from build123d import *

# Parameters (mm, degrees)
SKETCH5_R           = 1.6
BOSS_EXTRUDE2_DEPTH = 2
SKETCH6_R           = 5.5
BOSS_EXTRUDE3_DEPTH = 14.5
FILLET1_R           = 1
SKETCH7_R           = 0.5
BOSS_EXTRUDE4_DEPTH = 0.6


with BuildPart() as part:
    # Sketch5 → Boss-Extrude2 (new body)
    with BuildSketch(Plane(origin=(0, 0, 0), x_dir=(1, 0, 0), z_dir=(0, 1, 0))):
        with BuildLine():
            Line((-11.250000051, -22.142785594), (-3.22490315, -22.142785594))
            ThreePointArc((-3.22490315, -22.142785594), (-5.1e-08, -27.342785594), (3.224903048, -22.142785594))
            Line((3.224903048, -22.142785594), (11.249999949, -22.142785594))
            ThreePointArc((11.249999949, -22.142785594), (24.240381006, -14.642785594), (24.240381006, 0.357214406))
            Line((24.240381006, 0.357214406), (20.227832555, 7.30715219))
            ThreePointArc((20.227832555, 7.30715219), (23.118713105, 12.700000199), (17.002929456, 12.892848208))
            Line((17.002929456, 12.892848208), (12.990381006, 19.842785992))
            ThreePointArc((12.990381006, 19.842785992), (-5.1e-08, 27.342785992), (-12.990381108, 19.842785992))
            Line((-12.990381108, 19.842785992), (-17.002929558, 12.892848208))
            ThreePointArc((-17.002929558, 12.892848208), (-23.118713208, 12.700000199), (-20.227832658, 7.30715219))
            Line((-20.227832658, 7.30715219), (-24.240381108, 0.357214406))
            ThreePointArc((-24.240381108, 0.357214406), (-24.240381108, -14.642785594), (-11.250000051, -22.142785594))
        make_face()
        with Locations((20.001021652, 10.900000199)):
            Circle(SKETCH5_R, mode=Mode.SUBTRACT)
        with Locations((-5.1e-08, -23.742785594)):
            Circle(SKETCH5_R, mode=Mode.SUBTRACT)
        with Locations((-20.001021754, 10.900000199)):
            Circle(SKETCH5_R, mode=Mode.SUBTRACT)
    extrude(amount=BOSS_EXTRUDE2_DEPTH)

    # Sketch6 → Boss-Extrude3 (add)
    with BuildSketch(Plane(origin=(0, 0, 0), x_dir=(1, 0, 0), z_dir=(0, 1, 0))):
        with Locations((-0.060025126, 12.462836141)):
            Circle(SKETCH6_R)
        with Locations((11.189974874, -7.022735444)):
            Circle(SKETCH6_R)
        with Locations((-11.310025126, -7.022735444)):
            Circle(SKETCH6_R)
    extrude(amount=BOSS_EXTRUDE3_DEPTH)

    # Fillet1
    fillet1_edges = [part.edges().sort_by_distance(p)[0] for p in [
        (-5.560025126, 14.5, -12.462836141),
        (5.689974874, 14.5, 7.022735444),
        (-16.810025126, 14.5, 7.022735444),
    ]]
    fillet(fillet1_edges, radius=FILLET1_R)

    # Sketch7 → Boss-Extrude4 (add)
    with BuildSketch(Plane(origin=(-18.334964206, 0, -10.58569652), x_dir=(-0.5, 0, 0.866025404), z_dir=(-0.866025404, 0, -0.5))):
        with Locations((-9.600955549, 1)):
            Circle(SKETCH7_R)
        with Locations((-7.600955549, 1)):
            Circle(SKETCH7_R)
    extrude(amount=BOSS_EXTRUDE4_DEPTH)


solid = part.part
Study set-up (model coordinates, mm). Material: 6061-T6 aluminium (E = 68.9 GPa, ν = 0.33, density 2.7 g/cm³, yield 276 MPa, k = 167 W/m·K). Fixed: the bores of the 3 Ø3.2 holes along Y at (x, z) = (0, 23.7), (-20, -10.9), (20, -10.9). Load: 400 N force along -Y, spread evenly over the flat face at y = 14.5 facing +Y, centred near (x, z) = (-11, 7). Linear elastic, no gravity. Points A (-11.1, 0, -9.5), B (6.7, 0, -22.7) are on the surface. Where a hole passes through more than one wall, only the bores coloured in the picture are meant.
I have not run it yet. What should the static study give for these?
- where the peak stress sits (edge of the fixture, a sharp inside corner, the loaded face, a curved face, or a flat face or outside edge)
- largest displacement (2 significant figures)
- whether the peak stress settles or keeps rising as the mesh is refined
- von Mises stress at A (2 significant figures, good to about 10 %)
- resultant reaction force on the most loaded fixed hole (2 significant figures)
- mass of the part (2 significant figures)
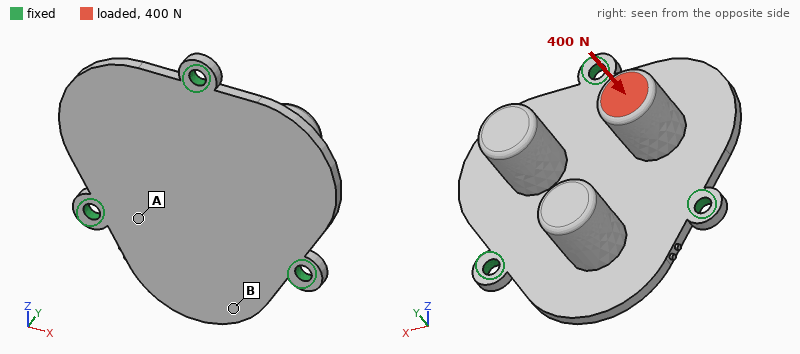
edge of the fixture
0.19 mm
keeps rising
37 MPa
210 N
20 g
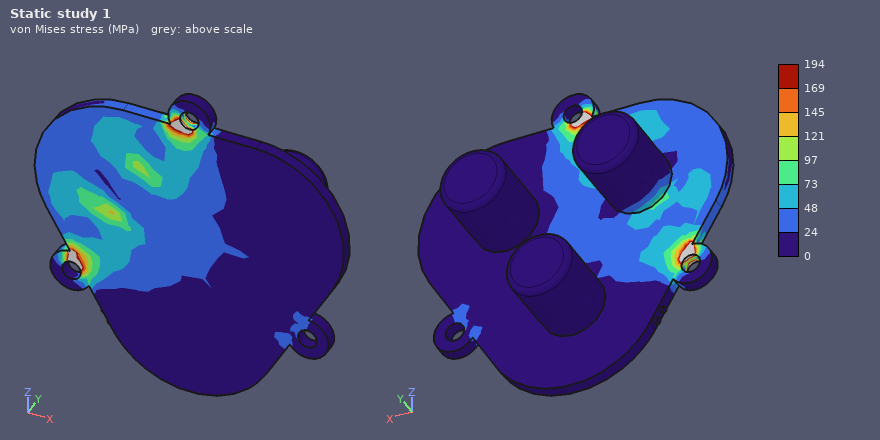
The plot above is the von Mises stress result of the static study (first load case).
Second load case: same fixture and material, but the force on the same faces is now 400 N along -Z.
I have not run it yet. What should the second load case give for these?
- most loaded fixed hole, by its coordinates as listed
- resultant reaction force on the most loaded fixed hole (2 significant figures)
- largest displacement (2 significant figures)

(0, 23.7)
260 N
0.20 mm
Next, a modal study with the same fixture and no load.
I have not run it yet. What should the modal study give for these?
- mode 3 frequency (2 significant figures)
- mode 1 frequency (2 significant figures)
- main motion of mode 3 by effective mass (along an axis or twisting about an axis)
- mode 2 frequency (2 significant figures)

3800 Hz
3100 Hz
along Y
3100 Hz
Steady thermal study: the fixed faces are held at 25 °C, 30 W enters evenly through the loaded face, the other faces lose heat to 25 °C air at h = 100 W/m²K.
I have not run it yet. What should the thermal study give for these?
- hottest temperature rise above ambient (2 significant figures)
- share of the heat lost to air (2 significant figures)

61 K
31 %
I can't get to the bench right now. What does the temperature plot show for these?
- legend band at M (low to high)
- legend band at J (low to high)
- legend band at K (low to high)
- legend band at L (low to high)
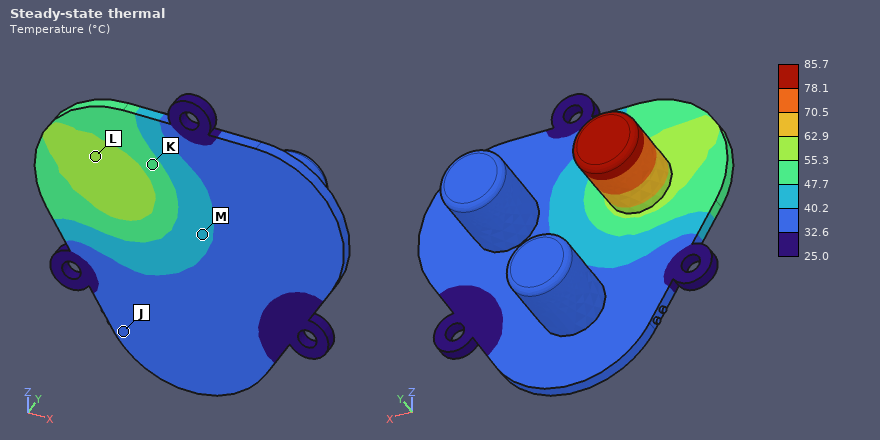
40.2 to 47.7 °C
32.6 to 40.2 °C
47.7 to 55.3 °C
55.3 to 62.9 °C
